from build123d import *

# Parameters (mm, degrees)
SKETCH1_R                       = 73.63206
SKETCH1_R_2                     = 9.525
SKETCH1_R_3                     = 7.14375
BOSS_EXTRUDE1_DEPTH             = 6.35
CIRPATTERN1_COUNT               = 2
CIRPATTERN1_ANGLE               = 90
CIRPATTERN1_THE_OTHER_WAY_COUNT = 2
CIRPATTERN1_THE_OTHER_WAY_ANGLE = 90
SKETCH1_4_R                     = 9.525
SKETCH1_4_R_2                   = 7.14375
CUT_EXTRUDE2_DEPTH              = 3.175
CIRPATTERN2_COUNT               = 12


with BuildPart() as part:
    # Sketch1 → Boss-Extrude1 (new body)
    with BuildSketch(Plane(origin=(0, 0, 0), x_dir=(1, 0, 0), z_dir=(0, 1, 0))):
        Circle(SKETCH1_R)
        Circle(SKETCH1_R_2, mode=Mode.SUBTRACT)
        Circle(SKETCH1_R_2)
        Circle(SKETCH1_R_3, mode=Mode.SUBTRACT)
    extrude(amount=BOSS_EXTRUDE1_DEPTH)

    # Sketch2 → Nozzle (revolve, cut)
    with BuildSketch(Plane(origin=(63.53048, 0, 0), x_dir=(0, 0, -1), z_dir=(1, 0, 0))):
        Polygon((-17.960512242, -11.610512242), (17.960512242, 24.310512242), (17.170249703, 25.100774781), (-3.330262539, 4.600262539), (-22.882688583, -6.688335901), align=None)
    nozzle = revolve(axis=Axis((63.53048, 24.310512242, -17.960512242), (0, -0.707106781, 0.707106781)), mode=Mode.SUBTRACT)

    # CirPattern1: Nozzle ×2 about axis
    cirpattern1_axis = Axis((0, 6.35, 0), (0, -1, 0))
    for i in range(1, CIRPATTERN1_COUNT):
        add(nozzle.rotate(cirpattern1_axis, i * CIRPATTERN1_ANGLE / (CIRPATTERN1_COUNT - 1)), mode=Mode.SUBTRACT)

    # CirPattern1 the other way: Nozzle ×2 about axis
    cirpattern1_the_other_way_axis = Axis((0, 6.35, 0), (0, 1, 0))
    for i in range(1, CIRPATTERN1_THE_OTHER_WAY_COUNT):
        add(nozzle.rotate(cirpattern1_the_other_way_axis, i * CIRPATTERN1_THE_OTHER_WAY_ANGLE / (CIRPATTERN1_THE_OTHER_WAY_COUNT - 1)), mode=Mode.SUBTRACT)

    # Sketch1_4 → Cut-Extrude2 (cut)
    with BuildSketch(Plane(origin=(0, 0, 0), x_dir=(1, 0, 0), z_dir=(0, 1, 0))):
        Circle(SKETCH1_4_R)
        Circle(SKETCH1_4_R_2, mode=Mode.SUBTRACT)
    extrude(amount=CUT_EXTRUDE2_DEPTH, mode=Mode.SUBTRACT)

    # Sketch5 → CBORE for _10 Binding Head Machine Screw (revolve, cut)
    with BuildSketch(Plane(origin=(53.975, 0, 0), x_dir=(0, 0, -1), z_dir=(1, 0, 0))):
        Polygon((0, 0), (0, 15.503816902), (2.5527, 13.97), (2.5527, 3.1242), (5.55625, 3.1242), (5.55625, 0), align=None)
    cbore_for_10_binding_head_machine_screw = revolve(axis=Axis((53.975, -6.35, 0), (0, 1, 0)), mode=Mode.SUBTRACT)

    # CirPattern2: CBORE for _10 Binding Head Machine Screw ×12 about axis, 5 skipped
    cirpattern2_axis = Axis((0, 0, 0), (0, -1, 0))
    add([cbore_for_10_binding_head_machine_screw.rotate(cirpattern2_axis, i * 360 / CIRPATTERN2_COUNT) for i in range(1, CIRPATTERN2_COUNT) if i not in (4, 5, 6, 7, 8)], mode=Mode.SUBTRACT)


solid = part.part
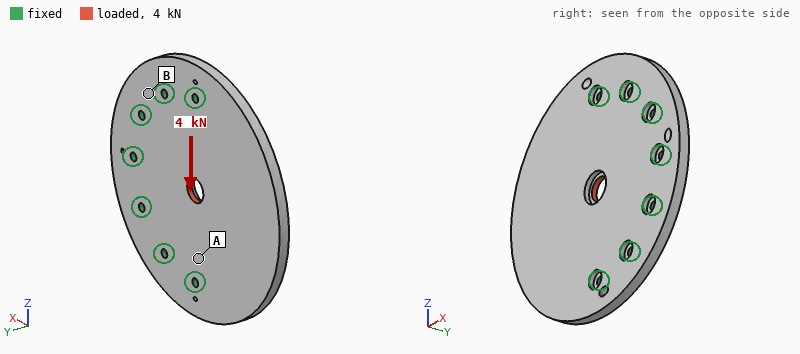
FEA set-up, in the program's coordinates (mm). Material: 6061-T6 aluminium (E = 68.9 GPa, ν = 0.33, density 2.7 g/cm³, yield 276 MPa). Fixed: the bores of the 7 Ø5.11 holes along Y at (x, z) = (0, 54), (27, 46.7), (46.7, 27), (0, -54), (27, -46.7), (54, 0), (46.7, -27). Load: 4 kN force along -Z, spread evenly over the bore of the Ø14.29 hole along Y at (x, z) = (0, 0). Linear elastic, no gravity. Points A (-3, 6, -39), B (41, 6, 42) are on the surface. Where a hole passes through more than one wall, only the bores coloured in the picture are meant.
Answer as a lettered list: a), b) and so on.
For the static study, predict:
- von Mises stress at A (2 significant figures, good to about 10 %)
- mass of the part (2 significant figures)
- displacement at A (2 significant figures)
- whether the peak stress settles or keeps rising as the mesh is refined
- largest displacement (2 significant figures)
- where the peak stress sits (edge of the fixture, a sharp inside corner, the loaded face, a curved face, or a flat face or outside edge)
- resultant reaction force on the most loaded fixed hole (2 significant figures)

a) 11 MPa
b) 280 g
c) 4.9 µm
d) keeps rising
e) 10 µm
f) edge of the fixture
g) 1.1 kN
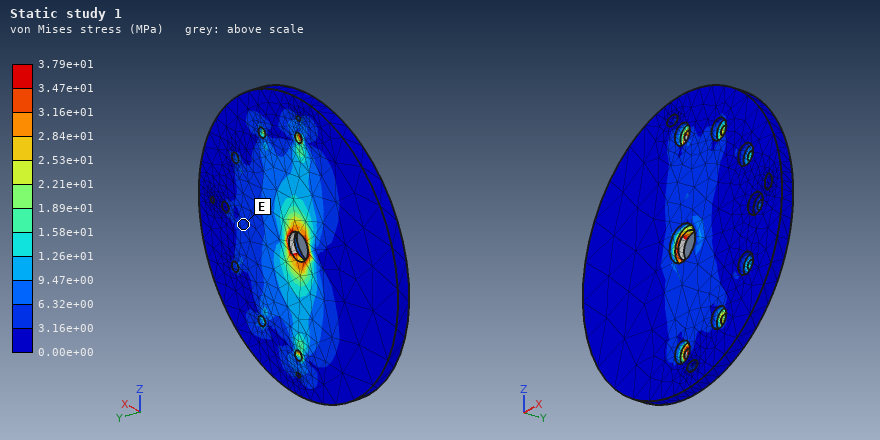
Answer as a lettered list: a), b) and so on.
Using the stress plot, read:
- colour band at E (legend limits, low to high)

a) 3.16e+00 to 6.32e+00 MPa
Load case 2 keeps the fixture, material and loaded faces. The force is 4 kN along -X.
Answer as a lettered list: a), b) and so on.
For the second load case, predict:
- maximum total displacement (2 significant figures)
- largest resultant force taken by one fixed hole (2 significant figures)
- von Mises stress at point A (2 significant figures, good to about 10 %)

a) 31 µm
b) 720 N
c) 6.1 MPa
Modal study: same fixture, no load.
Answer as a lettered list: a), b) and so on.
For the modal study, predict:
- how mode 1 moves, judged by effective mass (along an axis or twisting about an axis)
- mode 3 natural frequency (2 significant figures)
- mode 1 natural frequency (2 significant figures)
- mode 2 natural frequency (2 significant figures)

a) along Y
b) 3300 Hz
c) 840 Hz
d) 2200 Hz
